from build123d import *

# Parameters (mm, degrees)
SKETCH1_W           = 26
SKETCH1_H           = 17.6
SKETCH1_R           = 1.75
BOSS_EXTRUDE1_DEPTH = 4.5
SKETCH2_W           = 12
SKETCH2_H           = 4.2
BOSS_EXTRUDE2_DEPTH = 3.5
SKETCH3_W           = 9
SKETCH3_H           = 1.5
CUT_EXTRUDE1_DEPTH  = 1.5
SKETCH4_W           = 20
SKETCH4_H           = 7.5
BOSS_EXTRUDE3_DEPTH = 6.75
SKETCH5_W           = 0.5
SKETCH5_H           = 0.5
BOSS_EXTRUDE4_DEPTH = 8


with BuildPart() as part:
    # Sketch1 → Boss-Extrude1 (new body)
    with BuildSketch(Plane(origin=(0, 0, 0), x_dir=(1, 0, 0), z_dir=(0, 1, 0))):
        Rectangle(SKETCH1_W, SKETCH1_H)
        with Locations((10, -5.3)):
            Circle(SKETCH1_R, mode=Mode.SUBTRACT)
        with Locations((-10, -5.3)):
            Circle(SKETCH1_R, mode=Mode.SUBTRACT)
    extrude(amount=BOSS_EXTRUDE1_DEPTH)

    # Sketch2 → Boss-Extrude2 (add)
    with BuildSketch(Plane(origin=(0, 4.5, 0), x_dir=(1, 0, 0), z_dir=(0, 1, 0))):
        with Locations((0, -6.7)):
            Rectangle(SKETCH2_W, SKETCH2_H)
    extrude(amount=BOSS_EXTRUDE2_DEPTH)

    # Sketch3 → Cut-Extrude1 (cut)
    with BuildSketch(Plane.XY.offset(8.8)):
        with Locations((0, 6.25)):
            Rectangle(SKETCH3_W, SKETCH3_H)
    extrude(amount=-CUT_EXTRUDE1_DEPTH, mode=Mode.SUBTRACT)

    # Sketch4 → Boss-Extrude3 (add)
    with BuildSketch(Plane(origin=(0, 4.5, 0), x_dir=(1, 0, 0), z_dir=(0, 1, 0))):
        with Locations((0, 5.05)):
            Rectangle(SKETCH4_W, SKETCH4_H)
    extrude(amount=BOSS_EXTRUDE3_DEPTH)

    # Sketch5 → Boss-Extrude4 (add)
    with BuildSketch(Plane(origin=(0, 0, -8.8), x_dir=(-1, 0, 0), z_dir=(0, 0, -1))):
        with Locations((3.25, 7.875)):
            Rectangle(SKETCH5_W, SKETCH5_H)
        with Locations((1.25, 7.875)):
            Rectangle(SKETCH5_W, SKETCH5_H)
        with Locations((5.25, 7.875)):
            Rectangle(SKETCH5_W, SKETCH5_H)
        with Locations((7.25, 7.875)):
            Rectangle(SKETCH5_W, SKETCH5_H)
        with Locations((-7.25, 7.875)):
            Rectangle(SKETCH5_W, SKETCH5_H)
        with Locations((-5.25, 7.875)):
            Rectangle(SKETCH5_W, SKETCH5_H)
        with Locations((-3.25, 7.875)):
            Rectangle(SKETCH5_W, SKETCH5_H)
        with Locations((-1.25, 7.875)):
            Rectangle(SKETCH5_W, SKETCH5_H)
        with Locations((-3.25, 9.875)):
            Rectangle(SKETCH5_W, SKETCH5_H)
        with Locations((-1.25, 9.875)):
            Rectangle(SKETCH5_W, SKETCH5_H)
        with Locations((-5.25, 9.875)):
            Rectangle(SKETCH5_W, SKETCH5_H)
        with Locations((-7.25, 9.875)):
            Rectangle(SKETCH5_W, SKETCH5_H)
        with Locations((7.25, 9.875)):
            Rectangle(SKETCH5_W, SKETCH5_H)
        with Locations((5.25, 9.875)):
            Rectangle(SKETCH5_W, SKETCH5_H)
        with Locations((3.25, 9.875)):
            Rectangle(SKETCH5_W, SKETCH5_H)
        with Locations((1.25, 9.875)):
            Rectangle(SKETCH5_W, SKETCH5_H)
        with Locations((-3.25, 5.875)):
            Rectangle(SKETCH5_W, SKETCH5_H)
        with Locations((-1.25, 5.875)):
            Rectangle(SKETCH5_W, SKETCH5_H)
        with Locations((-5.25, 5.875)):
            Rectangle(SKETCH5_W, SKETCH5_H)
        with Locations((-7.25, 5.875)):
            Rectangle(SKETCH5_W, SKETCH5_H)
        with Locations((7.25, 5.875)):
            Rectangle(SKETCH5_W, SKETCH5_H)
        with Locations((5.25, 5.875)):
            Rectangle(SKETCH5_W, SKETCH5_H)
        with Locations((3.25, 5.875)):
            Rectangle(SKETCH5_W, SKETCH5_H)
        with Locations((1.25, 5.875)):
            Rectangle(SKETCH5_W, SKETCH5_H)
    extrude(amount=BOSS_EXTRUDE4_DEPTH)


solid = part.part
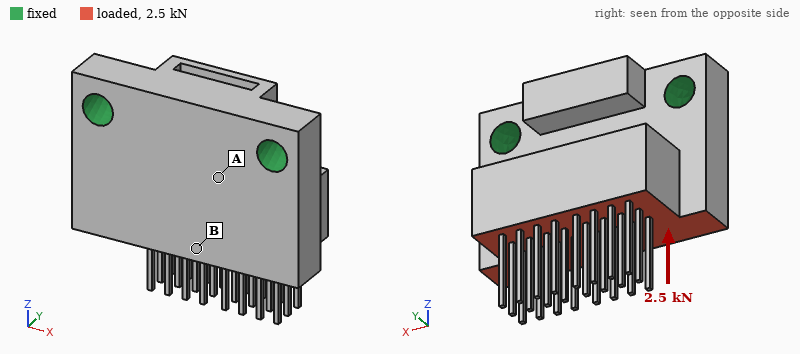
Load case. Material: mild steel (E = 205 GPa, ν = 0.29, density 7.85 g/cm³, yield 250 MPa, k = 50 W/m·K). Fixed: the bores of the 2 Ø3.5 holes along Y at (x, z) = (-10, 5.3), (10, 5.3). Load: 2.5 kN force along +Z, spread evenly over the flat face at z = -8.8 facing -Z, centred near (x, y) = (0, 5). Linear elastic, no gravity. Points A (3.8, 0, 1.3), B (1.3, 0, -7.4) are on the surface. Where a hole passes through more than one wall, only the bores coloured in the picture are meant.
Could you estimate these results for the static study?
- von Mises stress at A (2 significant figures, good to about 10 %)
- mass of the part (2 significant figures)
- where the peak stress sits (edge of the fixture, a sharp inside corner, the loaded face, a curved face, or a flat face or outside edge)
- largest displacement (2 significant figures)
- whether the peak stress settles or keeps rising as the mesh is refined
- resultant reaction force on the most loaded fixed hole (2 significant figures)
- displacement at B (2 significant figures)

49 MPa
25 g
edge of the fixture
34 µm
keeps rising
1.3 kN
14 µm
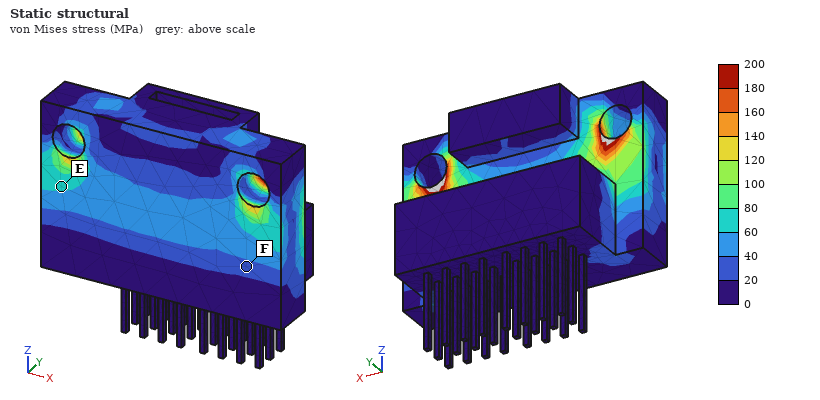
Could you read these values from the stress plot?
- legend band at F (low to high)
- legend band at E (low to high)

20 to 40 MPa
60 to 80 MPa
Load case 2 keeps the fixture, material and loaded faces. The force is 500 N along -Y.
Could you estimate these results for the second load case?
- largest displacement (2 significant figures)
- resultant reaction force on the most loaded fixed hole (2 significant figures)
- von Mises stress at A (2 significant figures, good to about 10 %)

24 µm
250 N
38 MPa
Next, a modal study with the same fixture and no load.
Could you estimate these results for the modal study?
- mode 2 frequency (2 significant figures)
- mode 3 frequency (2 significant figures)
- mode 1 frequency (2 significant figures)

6300 Hz
6300 Hz
6200 Hz
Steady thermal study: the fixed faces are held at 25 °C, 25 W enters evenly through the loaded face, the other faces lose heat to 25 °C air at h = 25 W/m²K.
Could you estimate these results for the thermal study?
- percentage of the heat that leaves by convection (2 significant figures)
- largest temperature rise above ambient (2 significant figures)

6.0 %
55 K
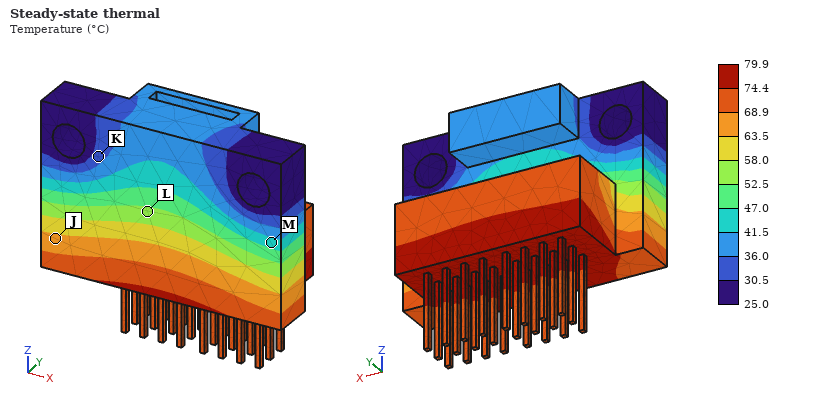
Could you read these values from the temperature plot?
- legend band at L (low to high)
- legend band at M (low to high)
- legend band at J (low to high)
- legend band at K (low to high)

52.5 to 58.0 °C
41.5 to 47.0 °C
63.5 to 68.9 °C
30.5 to 36.0 °C
